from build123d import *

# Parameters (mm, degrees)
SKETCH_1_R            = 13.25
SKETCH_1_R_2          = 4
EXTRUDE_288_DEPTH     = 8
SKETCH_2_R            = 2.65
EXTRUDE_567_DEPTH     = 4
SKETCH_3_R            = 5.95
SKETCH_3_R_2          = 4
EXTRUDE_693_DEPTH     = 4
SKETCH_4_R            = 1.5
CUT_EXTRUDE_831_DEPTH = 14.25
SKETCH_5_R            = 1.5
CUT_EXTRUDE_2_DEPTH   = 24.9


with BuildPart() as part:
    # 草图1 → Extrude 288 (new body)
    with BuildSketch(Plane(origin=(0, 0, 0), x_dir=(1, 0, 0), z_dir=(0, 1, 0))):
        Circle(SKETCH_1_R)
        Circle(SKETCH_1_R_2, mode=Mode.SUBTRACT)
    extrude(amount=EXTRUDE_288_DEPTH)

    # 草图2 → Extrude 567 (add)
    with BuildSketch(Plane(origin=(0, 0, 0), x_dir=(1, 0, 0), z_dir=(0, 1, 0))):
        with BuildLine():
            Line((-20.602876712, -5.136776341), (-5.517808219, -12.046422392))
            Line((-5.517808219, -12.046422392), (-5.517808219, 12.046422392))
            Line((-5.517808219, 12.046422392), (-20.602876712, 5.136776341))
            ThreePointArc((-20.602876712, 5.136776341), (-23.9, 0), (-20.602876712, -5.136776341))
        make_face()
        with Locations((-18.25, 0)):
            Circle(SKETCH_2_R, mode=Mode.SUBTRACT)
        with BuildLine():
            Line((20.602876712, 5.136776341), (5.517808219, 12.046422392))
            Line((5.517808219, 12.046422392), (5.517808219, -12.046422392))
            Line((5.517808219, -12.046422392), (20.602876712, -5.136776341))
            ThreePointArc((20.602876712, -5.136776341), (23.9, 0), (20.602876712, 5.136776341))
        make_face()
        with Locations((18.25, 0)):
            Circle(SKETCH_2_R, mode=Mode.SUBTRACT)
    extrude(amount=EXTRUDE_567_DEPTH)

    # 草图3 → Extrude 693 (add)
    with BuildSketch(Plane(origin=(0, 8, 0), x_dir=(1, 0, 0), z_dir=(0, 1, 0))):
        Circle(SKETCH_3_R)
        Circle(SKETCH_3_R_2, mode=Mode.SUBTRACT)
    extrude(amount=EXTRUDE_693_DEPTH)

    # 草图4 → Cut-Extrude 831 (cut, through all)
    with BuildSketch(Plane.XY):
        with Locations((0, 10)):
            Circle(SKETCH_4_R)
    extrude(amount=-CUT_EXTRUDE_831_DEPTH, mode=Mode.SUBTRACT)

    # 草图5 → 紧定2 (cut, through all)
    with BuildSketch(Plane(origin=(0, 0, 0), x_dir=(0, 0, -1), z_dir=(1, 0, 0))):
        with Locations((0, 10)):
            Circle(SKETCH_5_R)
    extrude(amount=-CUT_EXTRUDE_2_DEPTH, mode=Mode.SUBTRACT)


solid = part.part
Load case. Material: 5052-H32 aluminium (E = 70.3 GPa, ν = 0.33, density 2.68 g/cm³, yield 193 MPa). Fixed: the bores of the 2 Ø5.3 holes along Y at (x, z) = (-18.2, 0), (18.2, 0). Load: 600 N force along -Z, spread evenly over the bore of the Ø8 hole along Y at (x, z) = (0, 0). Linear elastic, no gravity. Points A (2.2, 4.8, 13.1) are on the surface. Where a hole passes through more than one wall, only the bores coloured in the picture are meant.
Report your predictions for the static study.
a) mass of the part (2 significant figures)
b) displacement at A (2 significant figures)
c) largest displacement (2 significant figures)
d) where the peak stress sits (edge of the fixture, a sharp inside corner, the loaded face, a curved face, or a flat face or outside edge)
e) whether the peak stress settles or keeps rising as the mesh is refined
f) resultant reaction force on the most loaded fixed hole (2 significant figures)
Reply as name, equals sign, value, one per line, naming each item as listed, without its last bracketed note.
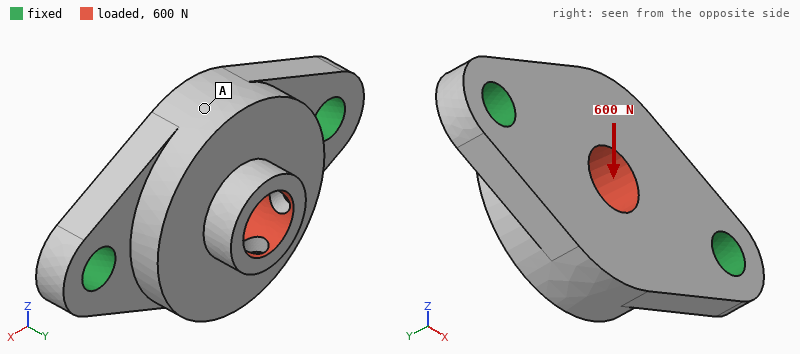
mass of the part = 14 g
displacement at A = 9.8 µm
largest displacement = 11 µm
where the peak stress sits = edge of the fixture
whether the peak stress settles or keeps rising as the mesh is refined = keeps rising
resultant reaction force on the most loaded fixed hole = 300 N
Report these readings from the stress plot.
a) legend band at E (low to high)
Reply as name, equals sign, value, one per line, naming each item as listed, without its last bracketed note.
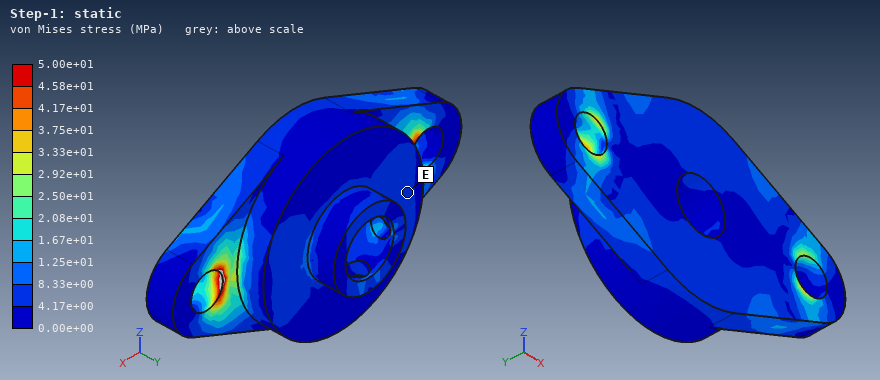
legend band at E = 4.17e+00 to 8.33e+00 MPa
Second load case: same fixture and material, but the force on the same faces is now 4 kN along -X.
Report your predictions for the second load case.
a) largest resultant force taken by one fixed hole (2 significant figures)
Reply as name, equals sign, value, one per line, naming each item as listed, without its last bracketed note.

largest resultant force taken by one fixed hole = 2.1 kN
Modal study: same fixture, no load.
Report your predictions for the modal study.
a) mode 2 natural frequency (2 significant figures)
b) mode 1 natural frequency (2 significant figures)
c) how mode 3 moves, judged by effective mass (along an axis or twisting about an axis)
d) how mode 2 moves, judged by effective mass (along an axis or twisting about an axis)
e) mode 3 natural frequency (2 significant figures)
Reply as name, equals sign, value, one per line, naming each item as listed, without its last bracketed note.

mode 2 natural frequency = 16 kHz
mode 1 natural frequency = 11 kHz
how mode 3 moves, judged by effective mass = along Z
how mode 2 moves, judged by effective mass = along Y
mode 3 natural frequency = 28 kHz
